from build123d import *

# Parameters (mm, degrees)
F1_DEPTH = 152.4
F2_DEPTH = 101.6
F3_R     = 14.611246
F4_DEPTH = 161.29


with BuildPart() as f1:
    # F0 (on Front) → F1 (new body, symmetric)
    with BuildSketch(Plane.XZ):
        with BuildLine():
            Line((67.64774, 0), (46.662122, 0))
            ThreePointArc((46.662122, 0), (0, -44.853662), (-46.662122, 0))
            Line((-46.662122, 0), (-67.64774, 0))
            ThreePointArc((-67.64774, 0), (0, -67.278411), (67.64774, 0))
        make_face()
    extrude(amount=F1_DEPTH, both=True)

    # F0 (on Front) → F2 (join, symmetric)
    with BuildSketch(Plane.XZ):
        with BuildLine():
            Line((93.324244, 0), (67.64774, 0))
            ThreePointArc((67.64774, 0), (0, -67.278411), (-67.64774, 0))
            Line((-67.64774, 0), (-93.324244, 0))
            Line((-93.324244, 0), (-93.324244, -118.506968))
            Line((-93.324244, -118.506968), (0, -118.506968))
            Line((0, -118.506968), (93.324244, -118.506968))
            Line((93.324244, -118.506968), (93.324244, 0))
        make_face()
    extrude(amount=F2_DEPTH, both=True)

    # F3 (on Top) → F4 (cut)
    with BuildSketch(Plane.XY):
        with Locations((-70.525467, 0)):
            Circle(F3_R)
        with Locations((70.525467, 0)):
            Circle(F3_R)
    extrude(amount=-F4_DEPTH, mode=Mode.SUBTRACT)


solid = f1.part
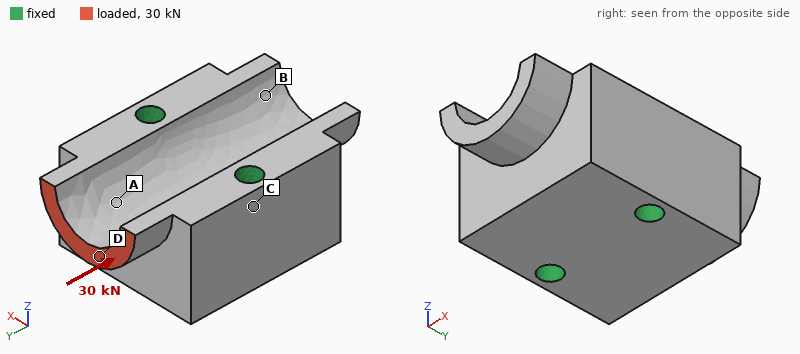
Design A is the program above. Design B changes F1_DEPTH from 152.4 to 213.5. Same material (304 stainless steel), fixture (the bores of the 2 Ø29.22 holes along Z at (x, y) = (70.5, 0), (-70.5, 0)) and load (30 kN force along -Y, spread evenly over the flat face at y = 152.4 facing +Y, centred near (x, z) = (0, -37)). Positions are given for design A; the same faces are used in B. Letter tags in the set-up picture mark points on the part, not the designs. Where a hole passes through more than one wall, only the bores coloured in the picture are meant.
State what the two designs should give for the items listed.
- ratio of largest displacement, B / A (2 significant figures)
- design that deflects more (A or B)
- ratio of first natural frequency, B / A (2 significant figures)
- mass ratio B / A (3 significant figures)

1.4
B
0.51
1.12
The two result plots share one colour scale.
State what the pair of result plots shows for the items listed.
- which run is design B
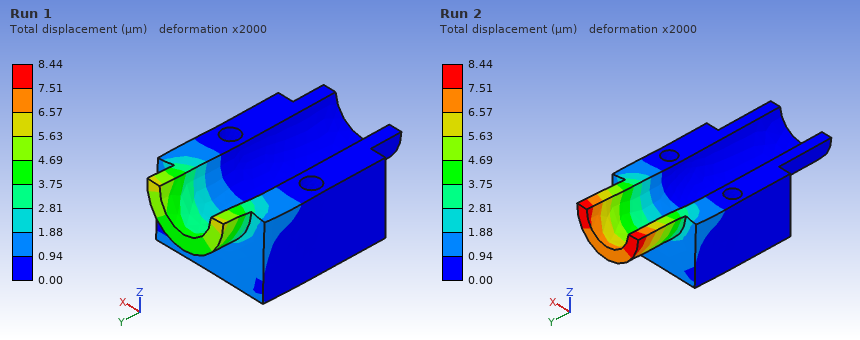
Run 2
